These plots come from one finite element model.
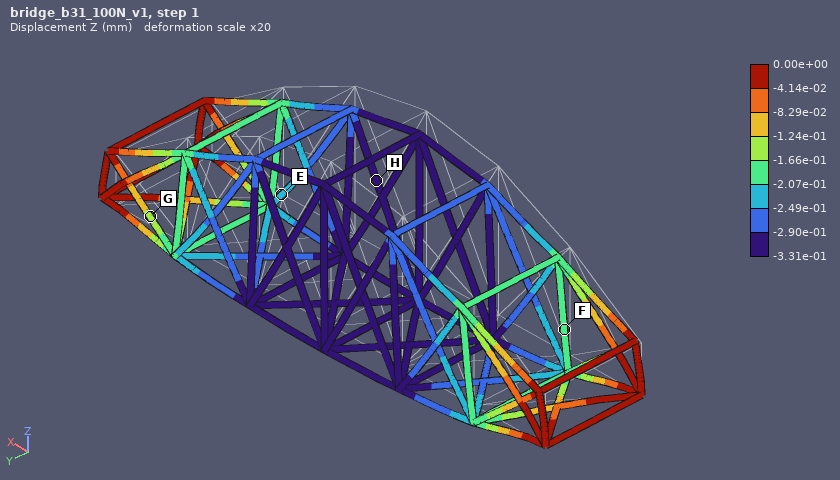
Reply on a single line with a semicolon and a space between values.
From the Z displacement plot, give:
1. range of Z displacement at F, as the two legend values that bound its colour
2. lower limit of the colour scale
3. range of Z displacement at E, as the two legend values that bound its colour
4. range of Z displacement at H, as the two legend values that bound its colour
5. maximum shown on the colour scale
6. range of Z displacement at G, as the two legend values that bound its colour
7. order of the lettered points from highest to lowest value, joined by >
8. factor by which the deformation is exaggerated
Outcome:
-2.07e-01 to -1.66e-01 mm; -3.31e-01 mm; -2.49e-01 to -2.07e-01 mm; -3.31e-01 to -2.90e-01 mm; 0.00e+00 mm; -1.66e-01 to -1.24e-01 mm; G > F > E > H; 20
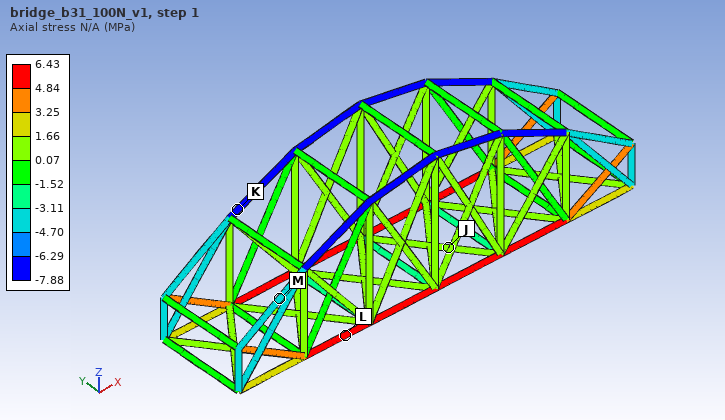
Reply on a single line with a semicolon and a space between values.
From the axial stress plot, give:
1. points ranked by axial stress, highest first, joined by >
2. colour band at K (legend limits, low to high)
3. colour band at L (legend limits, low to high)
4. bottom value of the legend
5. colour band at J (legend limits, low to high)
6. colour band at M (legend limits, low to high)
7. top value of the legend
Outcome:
L > J > M > K; -7.88 to -6.29 MPa; 4.84 to 6.43 MPa; -7.88 MPa; 0.07 to 1.66 MPa; -4.70 to -3.11 MPa; 6.43 MPa
